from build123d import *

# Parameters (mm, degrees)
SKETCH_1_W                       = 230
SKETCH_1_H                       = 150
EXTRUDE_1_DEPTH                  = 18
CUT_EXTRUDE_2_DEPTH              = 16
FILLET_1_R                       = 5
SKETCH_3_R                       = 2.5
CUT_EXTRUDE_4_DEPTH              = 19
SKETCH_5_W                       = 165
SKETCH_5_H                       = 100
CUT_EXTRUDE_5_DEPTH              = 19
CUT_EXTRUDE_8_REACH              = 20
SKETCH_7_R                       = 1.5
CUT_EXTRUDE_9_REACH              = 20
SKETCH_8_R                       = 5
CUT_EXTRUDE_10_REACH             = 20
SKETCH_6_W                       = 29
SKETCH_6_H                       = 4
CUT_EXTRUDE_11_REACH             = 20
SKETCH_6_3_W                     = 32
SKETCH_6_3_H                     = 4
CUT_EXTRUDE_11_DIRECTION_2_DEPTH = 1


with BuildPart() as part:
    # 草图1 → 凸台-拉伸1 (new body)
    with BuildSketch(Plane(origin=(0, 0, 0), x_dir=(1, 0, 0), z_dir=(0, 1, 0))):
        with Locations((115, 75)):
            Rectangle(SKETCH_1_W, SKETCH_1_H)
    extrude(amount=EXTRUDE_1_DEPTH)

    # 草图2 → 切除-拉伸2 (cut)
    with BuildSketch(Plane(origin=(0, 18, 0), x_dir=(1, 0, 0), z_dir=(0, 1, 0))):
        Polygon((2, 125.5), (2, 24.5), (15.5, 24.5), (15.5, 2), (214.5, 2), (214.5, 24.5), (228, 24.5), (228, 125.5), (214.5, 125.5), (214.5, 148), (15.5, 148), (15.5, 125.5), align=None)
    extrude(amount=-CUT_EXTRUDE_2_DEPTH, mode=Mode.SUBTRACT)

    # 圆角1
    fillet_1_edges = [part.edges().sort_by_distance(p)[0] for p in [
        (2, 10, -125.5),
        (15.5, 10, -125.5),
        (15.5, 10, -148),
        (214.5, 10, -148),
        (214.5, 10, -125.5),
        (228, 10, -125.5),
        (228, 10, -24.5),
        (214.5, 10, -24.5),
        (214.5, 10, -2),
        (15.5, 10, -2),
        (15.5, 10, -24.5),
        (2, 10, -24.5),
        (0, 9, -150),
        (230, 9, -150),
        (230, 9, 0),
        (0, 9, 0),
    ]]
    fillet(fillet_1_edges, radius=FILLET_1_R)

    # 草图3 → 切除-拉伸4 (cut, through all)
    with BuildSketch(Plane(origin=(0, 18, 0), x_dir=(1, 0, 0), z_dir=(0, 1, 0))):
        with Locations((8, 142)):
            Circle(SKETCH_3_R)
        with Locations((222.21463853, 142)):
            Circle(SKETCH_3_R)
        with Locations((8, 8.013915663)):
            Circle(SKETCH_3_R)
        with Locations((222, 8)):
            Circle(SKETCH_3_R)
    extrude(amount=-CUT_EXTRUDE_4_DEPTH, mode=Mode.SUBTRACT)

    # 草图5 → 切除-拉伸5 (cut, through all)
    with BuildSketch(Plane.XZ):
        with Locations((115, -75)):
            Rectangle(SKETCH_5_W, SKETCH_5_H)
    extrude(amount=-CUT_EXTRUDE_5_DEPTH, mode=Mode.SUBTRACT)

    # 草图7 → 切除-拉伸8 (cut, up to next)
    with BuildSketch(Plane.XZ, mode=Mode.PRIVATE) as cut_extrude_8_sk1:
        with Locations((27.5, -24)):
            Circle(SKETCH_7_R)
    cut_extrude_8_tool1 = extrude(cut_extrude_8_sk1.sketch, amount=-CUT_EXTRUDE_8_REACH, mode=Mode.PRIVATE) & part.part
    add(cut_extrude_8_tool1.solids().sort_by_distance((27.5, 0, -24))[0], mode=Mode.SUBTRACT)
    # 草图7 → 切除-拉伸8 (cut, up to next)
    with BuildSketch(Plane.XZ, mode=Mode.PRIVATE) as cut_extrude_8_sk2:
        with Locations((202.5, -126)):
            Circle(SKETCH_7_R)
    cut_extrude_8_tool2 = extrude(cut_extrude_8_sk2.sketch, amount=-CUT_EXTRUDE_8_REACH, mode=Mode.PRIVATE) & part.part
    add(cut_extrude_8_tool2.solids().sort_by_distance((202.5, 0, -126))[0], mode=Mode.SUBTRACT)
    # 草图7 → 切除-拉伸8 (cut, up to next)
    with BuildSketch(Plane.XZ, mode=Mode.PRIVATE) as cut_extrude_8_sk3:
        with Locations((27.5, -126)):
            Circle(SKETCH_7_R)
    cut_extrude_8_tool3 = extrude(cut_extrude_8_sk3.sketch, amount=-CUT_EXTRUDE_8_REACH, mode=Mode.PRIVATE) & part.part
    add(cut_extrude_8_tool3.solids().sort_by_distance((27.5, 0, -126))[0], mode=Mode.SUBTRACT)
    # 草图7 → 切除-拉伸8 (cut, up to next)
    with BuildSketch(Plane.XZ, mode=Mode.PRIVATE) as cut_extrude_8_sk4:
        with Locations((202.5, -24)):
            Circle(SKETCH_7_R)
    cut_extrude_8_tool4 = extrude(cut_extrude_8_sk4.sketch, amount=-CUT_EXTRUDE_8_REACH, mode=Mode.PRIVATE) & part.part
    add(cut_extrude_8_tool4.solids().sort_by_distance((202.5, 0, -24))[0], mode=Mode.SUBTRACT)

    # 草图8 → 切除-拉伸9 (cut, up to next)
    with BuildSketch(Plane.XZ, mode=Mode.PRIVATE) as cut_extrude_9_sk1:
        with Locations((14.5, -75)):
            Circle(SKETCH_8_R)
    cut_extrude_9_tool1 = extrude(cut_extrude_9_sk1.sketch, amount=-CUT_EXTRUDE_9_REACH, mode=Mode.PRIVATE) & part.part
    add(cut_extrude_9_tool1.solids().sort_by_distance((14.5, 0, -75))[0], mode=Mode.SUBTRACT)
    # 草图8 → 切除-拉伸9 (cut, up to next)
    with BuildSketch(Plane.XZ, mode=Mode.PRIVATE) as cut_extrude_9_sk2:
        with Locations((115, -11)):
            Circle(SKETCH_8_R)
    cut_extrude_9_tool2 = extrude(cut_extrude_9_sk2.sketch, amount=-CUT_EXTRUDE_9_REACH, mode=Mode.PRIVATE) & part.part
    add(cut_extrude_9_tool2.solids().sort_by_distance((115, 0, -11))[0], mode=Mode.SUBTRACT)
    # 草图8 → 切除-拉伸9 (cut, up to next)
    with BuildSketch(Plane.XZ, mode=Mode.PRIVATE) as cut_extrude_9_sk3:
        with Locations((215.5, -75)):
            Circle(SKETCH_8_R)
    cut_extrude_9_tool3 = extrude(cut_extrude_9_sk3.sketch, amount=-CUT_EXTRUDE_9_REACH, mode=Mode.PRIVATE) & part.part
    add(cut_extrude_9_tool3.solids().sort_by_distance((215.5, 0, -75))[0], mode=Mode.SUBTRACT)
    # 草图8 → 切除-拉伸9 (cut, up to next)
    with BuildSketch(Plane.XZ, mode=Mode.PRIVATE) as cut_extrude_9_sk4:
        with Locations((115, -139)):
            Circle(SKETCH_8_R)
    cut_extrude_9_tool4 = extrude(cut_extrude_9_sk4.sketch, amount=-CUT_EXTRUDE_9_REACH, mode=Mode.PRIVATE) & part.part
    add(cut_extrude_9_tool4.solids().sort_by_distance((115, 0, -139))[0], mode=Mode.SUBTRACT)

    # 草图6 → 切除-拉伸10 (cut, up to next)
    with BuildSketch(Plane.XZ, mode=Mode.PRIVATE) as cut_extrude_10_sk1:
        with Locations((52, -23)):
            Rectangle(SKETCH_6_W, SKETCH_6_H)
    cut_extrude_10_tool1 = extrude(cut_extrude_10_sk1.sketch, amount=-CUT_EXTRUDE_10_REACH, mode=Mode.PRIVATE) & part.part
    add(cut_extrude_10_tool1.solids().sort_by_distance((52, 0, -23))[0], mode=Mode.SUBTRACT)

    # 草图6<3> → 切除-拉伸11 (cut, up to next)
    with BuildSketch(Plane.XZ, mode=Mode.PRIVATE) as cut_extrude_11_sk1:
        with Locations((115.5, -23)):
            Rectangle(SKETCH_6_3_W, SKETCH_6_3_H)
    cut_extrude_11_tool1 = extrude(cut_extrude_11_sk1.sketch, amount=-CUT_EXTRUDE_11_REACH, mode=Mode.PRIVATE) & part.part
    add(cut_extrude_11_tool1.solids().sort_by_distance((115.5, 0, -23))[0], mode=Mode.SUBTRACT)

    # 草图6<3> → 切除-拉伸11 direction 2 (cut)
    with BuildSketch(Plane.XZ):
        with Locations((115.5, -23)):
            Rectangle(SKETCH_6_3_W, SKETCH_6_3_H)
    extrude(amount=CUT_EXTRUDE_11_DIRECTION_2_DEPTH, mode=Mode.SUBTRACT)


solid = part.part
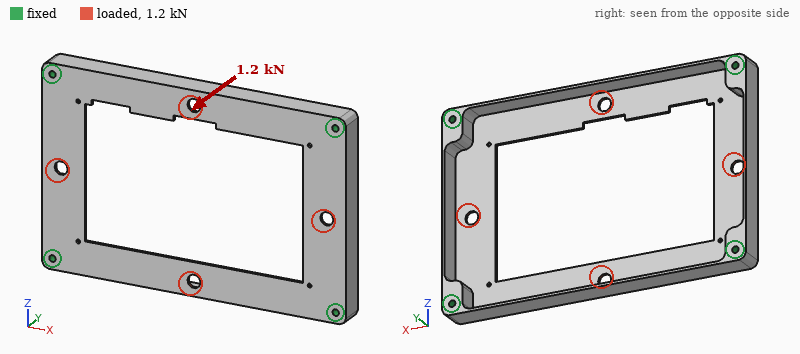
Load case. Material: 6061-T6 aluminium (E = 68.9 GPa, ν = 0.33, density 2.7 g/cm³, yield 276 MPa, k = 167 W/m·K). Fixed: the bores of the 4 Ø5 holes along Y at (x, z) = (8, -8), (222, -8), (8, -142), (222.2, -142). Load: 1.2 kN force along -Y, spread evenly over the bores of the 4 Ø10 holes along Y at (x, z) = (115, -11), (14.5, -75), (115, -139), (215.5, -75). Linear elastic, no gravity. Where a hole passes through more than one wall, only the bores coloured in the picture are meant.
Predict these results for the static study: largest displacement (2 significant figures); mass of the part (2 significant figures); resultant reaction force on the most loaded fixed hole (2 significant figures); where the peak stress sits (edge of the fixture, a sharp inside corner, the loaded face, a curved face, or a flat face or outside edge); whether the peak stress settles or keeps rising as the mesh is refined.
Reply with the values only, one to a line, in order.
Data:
1.1 mm
210 g
310 N
a sharp inside corner
keeps rising
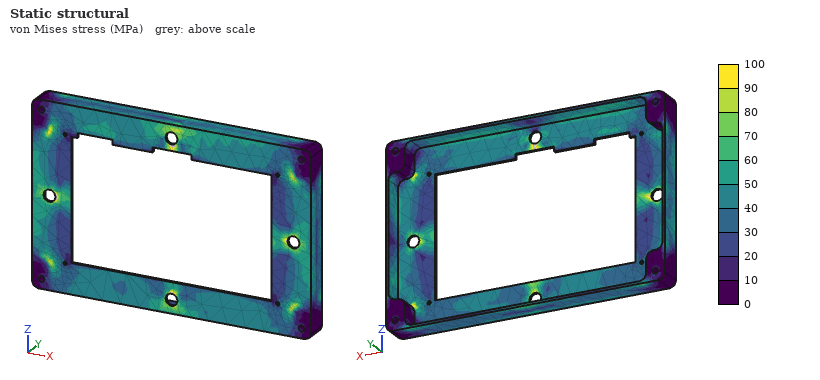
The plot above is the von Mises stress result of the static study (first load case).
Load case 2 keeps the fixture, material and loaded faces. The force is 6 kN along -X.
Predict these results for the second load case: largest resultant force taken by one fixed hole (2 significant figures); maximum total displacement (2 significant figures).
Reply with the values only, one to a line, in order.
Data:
1.5 kN
84 µm
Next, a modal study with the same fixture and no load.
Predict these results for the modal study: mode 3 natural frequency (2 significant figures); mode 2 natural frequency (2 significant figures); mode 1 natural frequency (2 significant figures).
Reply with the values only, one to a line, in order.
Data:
1400 Hz
880 Hz
840 Hz
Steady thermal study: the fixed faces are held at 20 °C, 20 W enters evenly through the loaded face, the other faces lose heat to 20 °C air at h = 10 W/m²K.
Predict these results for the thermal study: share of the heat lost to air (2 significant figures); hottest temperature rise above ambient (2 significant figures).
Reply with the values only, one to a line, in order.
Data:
18 %
19 K
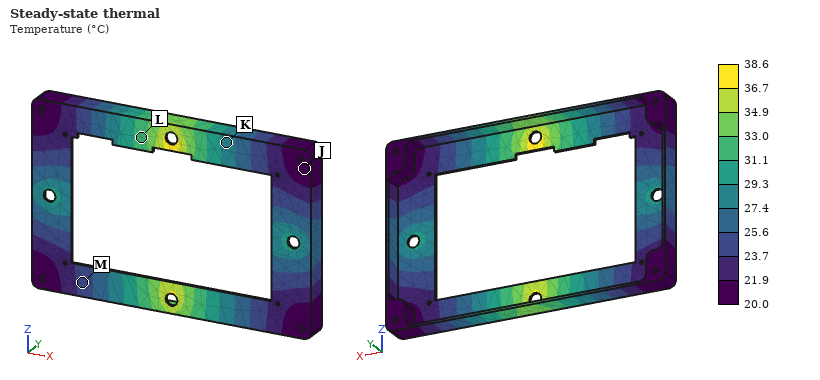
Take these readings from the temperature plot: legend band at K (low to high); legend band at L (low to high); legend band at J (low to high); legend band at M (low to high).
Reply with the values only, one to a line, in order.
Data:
27.4 to 29.3 °C
31.1 to 33.0 °C
20.0 to 21.9 °C
23.7 to 25.6 °C
